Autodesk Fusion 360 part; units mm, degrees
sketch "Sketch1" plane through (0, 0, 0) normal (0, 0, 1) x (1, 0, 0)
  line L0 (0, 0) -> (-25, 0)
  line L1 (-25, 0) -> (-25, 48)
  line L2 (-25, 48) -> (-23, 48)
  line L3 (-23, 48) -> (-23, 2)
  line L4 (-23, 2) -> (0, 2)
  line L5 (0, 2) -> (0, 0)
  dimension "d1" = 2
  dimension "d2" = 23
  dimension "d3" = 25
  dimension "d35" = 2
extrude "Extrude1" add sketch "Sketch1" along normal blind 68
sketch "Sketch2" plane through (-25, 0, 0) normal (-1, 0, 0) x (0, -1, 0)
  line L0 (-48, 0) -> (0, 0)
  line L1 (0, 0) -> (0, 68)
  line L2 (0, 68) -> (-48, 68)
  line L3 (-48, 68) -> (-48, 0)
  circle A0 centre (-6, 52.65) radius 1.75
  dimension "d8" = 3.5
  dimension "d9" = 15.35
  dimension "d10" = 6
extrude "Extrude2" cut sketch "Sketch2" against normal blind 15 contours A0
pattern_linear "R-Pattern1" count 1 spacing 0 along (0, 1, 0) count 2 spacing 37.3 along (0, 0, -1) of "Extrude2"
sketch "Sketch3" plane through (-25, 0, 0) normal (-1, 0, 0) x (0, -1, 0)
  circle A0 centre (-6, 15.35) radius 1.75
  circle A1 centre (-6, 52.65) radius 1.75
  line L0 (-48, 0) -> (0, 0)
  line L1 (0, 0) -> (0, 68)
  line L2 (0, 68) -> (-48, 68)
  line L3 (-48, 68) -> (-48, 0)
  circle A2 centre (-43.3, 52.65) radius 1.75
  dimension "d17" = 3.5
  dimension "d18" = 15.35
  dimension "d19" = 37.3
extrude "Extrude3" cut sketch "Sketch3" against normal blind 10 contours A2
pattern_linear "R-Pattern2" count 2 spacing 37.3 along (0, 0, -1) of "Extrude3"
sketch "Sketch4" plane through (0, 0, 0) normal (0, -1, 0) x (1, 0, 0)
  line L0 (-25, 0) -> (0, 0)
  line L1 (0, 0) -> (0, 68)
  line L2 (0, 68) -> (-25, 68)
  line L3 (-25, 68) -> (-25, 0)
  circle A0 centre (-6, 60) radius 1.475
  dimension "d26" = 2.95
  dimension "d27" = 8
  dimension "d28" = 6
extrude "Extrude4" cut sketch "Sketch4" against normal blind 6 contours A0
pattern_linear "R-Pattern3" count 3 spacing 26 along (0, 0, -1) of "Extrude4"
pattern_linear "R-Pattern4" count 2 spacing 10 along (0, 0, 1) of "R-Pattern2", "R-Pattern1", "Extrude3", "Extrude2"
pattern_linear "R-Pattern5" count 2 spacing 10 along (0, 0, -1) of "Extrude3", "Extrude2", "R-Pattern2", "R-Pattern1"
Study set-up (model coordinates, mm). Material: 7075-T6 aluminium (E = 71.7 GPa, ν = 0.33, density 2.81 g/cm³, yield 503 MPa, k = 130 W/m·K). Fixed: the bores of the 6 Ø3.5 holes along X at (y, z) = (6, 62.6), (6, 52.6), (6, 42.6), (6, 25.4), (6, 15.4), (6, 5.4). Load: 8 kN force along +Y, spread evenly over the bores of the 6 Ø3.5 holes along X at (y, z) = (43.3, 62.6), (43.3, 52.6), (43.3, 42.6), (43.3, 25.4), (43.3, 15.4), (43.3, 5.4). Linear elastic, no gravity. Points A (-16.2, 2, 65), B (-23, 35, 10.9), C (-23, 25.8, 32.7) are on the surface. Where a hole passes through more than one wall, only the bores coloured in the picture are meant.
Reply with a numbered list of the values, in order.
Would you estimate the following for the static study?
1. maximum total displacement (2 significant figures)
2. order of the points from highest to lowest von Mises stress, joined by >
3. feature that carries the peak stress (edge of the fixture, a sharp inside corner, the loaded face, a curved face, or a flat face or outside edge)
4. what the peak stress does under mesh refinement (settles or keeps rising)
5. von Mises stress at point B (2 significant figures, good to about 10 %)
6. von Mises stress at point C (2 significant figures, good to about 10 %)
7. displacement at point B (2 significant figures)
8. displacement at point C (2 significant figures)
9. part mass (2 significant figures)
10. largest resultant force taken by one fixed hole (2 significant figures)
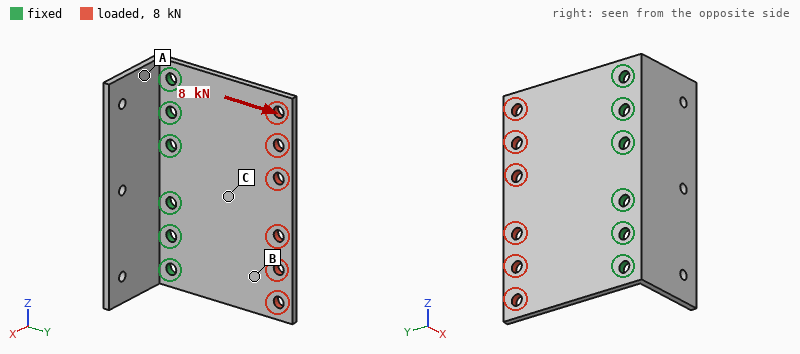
1. 39 µm
2. B > C > A
3. edge of the fixture
4. keeps rising
5. 67 MPa
6. 46 MPa
7. 26 µm
8. 15 µm
9. 26 g
10. 1.5 kN
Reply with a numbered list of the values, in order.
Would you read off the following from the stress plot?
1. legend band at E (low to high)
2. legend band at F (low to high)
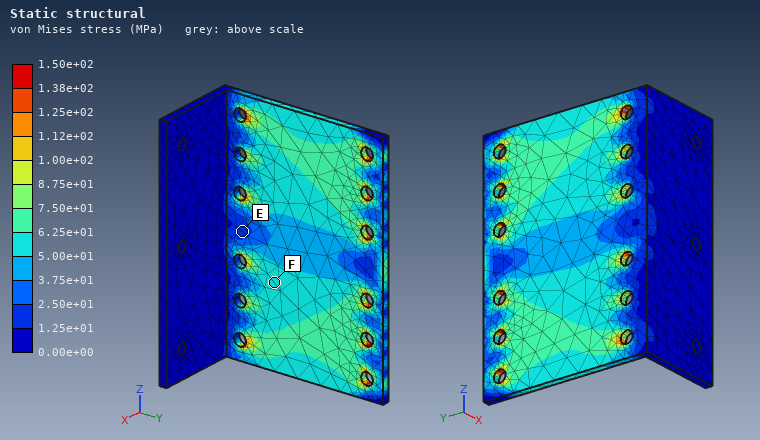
1. 1.25e+01 to 2.50e+01 MPa
2. 5.00e+01 to 6.25e+01 MPa
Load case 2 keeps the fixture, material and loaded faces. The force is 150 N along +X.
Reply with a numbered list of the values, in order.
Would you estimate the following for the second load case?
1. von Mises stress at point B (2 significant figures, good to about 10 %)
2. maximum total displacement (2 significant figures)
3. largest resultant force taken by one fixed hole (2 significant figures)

1. 27 MPa
2. 0.83 mm
3. 50 N
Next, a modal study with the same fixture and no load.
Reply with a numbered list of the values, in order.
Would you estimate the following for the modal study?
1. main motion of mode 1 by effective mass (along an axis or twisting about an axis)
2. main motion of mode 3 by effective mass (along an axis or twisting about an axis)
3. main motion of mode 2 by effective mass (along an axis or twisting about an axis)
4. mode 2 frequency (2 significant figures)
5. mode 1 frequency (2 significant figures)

1. along X
2. along Y
3. twisting about Y
4. 1700 Hz
5. 1000 Hz
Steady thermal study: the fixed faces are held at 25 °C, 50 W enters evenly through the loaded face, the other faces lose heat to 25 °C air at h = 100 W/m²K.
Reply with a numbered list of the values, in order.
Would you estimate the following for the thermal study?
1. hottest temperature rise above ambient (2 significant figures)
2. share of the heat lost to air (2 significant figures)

1. 79 K
2. 44 %
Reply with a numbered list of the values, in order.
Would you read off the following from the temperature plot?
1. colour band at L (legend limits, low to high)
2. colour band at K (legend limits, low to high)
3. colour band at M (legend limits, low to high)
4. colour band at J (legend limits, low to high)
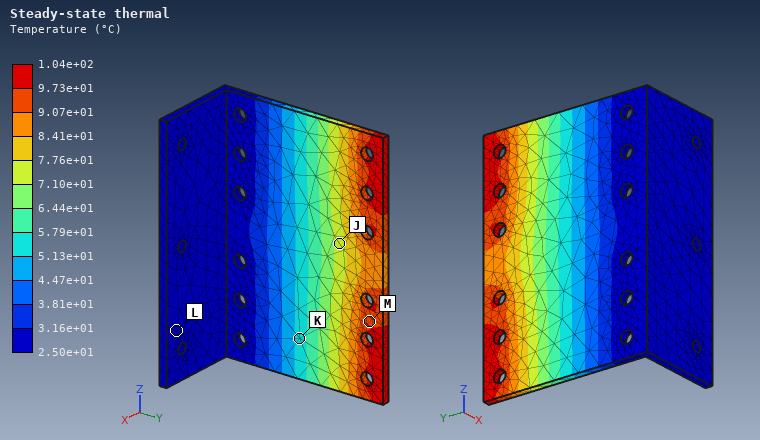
1. 2.50e+01 to 3.16e+01 °C
2. 5.13e+01 to 5.79e+01 °C
3. 9.07e+01 to 9.73e+01 °C
4. 7.10e+01 to 7.76e+01 °C
